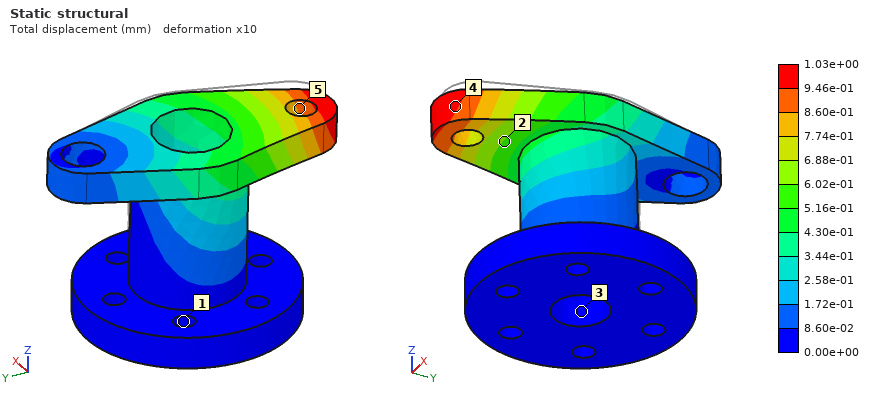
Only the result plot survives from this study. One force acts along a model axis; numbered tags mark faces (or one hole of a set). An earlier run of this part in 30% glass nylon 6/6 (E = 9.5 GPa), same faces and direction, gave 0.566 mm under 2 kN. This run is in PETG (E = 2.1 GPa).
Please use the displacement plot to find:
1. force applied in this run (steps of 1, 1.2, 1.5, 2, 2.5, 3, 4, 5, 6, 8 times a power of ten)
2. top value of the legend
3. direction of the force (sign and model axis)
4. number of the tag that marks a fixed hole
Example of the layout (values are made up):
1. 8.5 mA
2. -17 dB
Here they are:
1. 800 N
2. 1.03e+00 mm
3. -X
4. 1
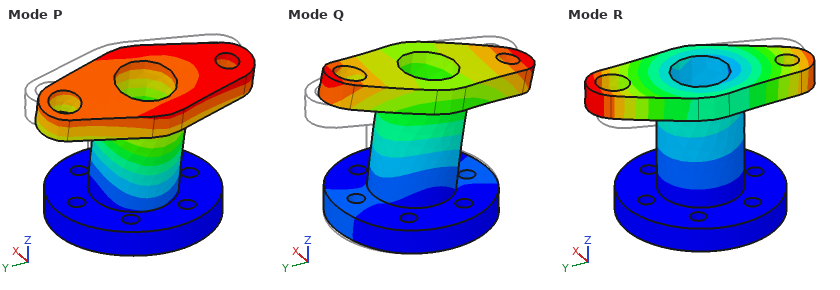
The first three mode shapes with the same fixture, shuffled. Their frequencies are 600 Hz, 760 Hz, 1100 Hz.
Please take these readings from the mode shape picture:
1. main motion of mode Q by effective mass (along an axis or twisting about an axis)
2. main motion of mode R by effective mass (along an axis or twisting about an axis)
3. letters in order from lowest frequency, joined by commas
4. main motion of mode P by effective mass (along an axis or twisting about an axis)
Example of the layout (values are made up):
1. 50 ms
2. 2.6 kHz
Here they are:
1. along Y
2. twisting about Z
3. Q, P, R
4. along X
